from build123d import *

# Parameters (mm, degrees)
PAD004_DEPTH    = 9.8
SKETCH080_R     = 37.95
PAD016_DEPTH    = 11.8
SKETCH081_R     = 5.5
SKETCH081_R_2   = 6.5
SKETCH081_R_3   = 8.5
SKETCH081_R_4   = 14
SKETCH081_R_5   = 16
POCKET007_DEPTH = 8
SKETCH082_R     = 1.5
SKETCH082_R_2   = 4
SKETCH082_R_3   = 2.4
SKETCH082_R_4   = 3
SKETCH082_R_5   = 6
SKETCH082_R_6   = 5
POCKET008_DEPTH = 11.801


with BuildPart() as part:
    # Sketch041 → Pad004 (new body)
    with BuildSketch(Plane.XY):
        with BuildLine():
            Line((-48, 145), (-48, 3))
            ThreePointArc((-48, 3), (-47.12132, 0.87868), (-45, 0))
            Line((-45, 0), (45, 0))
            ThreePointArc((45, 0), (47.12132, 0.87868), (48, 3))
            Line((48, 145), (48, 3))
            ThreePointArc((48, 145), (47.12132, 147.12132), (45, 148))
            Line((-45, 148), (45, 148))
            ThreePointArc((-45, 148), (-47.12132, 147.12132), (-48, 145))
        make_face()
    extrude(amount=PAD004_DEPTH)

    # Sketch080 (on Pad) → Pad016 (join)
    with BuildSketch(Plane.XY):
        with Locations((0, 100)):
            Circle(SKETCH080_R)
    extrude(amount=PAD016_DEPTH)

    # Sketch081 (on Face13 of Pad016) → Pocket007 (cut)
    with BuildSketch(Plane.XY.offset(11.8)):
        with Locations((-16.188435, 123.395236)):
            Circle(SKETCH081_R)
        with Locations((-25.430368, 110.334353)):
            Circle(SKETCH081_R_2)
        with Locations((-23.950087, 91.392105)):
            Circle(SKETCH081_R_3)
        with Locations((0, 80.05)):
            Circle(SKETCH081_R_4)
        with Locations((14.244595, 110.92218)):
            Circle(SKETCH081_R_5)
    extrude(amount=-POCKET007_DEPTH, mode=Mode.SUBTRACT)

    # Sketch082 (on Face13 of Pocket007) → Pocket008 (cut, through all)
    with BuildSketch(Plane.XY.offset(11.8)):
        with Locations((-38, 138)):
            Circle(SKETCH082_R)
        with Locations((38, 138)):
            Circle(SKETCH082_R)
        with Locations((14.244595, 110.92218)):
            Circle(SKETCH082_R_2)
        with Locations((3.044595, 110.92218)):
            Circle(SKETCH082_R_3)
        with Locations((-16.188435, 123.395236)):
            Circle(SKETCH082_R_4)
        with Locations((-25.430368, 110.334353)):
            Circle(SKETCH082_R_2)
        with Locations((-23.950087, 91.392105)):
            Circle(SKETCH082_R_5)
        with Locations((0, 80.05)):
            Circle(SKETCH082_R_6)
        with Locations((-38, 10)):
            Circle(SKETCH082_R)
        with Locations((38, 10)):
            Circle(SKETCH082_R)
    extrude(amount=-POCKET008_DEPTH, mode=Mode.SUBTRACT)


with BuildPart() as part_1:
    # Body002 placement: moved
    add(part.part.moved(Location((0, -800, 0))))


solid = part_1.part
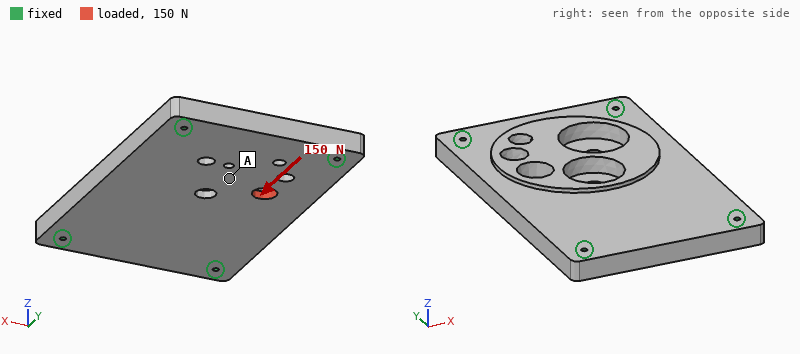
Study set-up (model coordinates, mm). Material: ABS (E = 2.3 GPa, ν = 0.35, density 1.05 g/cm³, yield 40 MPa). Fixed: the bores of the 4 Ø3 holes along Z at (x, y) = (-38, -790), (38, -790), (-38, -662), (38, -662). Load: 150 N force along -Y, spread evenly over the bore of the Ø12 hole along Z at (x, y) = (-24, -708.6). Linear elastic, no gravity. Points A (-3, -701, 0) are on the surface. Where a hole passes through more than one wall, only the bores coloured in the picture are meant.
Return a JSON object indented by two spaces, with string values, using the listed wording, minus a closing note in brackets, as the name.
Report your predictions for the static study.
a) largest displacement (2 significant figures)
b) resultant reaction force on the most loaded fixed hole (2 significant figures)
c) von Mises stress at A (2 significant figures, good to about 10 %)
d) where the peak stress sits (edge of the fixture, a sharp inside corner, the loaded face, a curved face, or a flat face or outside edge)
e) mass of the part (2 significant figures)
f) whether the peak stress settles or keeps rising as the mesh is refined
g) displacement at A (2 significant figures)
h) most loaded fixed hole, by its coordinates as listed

{
  "largest displacement": "12 µm",
  "resultant reaction force on the most loaded fixed hole": "62 N",
  "von Mises stress at A": "0.16 MPa",
  "where the peak stress sits": "a sharp inside corner",
  "mass of the part": "140 g",
  "whether the peak stress settles or keeps rising as the mesh is refined": "keeps rising",
  "displacement at A": "5.3 µm",
  "most loaded fixed hole, by its coordinates as listed": "(-38, -662)"
}
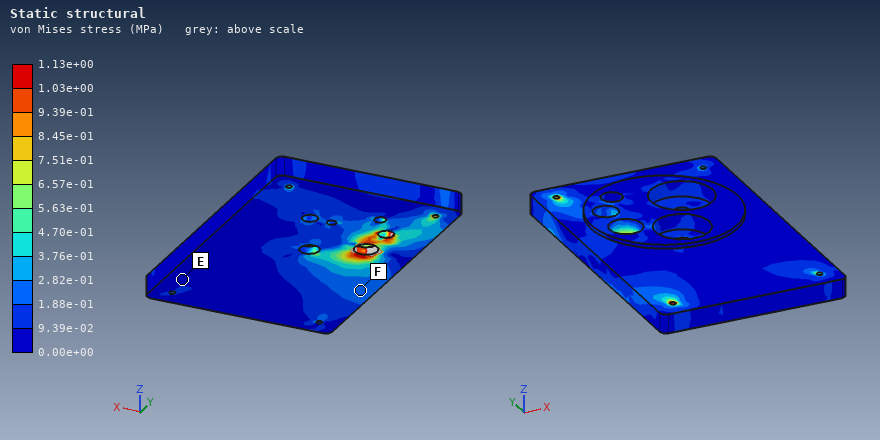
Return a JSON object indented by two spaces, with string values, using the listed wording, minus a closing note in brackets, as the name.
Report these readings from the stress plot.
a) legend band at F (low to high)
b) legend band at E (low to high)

{
  "legend band at F": "1.88e-01 to 2.82e-01 MPa",
  "legend band at E": "0.00e+00 to 9.39e-02 MPa"
}
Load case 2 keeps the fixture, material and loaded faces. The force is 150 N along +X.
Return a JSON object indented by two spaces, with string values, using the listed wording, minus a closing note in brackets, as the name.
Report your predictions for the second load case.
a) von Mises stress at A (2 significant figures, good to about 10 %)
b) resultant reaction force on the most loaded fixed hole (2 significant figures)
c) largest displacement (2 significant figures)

{
  "von Mises stress at A": "0.45 MPa",
  "resultant reaction force on the most loaded fixed hole": "49 N",
  "largest displacement": "21 µm"
}
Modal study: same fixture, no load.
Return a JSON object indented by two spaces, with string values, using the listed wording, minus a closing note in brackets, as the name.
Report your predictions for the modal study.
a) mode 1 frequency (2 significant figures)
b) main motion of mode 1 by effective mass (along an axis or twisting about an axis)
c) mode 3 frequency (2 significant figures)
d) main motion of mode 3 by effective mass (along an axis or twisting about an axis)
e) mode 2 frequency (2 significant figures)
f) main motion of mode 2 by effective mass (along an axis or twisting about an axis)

{
  "mode 1 frequency": "680 Hz",
  "main motion of mode 1 by effective mass": "along Z",
  "mode 3 frequency": "1700 Hz",
  "main motion of mode 3 by effective mass": "twisting about X",
  "mode 2 frequency": "1000 Hz",
  "main motion of mode 2 by effective mass": "twisting about Y"
}
